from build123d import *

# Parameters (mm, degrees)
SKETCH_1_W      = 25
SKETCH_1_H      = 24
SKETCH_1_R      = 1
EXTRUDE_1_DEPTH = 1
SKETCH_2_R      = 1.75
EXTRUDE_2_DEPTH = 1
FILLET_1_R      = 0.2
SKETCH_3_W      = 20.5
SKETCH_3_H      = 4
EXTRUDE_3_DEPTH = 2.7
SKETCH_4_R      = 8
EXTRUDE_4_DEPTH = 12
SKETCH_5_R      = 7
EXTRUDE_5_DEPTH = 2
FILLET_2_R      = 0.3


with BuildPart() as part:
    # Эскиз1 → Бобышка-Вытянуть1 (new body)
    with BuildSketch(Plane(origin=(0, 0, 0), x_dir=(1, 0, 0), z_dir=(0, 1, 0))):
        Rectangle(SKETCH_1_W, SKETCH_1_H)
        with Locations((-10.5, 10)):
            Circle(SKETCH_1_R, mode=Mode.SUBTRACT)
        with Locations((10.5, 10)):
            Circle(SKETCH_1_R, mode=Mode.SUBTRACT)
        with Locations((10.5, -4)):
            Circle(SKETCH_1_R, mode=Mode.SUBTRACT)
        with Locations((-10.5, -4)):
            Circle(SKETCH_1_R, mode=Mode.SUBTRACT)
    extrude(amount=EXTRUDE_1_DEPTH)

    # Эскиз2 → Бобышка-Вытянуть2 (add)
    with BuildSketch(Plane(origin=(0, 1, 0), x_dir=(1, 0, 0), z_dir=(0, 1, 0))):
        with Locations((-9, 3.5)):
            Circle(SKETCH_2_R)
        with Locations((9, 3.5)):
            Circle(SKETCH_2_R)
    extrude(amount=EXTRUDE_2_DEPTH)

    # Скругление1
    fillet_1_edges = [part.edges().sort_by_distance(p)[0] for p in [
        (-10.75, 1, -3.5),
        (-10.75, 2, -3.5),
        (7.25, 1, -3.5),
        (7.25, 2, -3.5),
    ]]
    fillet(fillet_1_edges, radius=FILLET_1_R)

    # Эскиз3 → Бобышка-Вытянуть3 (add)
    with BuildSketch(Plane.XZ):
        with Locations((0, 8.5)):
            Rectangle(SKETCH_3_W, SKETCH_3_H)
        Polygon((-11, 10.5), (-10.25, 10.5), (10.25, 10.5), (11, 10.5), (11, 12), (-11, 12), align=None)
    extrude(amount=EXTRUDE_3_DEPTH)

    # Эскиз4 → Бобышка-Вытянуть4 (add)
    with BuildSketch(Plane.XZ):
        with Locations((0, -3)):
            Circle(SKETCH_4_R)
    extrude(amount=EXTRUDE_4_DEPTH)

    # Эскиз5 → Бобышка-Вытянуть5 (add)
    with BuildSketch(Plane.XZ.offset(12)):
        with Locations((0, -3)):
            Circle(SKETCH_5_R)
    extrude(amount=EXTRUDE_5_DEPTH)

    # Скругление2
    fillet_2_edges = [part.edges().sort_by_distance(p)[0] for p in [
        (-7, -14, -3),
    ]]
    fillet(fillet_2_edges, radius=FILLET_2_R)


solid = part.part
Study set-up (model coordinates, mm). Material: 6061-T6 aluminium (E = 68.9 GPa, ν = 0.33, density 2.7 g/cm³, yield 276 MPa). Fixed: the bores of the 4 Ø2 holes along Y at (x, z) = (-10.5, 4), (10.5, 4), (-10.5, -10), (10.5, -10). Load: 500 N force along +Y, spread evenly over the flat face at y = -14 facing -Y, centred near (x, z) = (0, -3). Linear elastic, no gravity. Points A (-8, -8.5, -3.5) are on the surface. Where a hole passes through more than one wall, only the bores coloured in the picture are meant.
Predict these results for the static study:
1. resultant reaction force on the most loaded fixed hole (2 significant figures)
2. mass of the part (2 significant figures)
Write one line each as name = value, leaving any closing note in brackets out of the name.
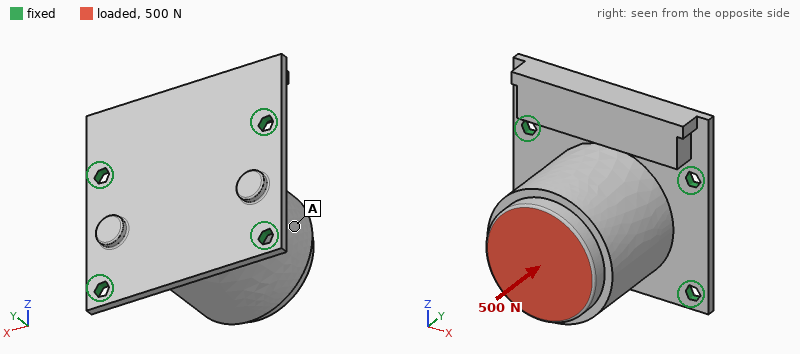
resultant reaction force on the most loaded fixed hole = 140 N
mass of the part = 9.8 g
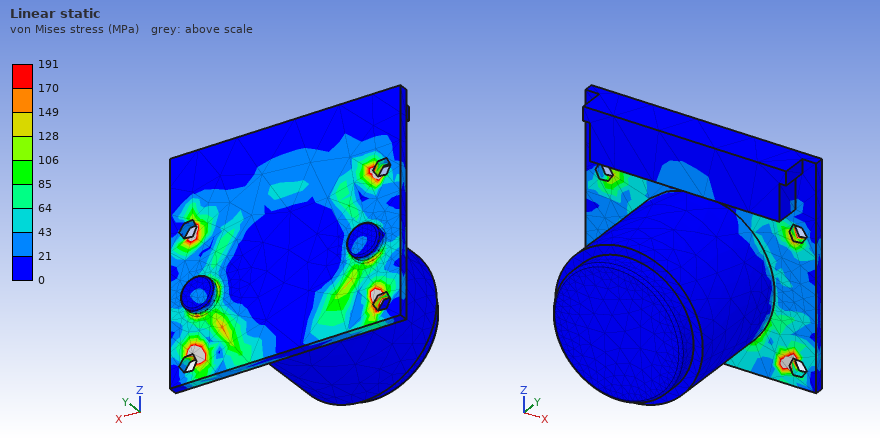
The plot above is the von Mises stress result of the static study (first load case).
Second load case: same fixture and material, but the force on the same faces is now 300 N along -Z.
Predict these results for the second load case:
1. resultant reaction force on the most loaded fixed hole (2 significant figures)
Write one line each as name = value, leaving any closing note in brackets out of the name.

resultant reaction force on the most loaded fixed hole = 210 N
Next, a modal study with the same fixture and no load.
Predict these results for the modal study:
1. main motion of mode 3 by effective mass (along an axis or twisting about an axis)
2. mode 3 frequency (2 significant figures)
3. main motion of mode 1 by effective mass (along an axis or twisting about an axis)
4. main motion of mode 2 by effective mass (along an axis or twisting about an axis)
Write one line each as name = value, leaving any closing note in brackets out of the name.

main motion of mode 3 by effective mass = along Y
mode 3 frequency = 8000 Hz
main motion of mode 1 by effective mass = along Z
main motion of mode 2 by effective mass = along X
